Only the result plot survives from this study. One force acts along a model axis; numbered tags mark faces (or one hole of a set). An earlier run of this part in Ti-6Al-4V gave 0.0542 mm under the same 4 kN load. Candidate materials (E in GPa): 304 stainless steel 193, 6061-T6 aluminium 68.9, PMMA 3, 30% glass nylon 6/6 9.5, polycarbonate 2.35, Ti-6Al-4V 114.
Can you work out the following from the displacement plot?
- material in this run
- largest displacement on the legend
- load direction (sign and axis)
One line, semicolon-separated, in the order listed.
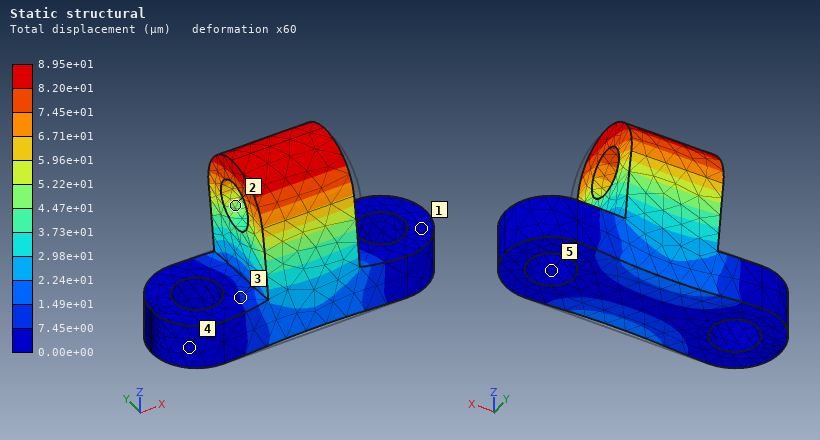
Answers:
6061-T6 aluminium; 8.95e+01 µm; +Y
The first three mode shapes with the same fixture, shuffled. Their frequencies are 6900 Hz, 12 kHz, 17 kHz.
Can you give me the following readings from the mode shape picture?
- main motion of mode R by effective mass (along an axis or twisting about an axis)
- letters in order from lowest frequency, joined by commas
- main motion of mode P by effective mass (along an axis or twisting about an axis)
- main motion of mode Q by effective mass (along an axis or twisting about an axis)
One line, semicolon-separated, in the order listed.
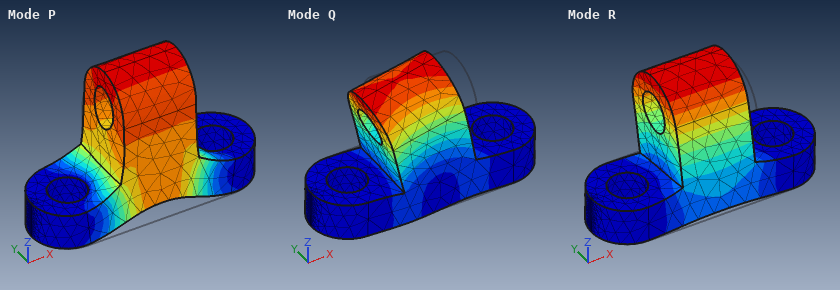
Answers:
along Y; R, Q, P; along Z; along X
